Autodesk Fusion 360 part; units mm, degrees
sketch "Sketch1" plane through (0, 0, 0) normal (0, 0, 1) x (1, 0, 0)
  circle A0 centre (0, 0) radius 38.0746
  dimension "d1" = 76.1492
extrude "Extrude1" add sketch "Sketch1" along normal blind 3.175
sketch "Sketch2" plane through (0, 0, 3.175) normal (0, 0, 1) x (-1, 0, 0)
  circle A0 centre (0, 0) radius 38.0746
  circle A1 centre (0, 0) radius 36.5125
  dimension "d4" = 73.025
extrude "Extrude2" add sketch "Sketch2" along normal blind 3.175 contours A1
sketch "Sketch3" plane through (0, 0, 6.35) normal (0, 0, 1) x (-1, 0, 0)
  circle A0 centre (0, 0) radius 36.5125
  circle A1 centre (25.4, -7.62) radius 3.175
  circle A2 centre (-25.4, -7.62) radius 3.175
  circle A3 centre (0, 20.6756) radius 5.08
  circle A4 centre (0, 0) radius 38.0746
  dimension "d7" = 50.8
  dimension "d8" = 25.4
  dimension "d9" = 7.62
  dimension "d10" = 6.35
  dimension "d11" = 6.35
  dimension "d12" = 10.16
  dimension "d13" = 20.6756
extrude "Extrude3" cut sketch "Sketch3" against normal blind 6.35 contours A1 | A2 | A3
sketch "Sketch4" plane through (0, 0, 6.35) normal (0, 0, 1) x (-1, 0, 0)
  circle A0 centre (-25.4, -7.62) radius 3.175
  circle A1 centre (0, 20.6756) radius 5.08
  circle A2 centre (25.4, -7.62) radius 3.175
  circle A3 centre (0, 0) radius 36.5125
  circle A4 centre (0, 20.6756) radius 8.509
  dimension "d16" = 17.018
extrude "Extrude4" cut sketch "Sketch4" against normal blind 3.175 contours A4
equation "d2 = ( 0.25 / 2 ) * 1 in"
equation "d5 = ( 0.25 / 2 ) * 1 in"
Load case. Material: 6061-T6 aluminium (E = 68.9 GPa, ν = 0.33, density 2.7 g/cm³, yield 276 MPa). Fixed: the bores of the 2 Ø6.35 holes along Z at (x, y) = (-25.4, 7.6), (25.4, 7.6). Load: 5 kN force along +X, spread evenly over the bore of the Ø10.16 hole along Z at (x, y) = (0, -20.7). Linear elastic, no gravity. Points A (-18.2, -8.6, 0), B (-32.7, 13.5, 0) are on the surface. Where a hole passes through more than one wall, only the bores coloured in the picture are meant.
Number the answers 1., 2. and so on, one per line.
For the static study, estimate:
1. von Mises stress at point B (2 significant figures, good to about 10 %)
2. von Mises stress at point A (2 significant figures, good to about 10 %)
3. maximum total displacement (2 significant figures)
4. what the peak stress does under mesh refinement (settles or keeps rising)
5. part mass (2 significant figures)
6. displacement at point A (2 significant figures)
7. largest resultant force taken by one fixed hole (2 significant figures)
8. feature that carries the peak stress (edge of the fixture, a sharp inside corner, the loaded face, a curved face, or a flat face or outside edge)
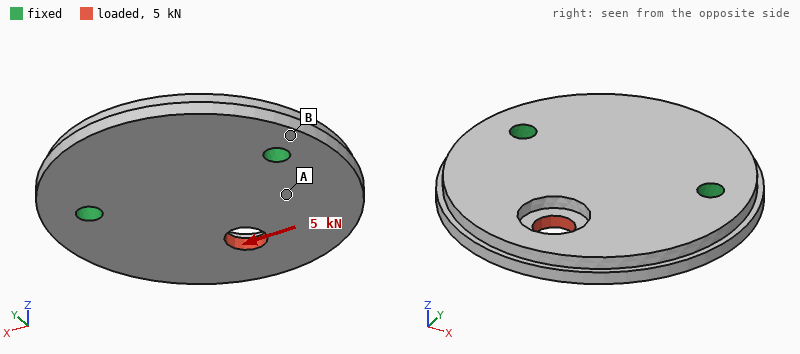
1. 13 MPa
2. 28 MPa
3. 31 µm
4. keeps rising
5. 71 g
6. 12 µm
7. 3.6 kN
8. a sharp inside corner
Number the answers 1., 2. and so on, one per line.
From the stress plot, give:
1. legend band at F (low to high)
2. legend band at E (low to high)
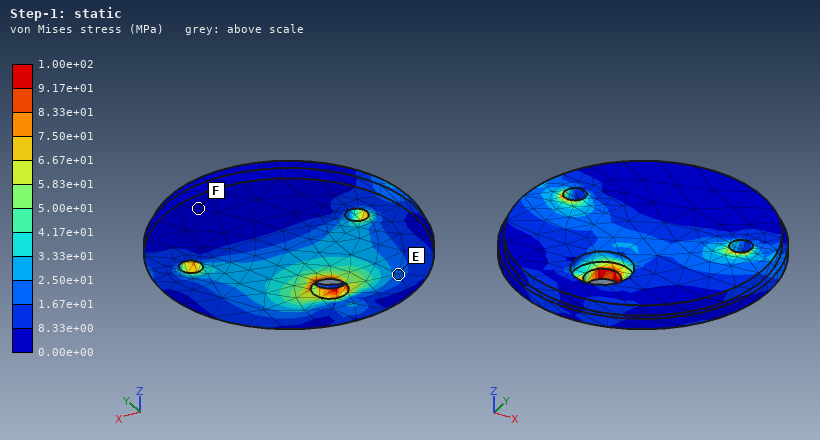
1. 0.00e+00 to 8.33e+00 MPa
2. 1.67e+01 to 2.50e+01 MPa
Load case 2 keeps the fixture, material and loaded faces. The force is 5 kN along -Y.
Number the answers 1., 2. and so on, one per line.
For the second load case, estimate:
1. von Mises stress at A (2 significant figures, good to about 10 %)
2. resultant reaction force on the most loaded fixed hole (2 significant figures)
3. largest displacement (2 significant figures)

1. 30 MPa
2. 2.6 kN
3. 84 µm
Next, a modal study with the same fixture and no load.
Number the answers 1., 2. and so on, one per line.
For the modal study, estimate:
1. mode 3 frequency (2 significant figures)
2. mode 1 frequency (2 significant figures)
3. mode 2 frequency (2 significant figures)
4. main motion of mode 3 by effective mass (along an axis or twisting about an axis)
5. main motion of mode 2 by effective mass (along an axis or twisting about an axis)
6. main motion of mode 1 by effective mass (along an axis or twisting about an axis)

1. 6700 Hz
2. 3000 Hz
3. 6100 Hz
4. twisting about Y
5. along Z
6. along Z
